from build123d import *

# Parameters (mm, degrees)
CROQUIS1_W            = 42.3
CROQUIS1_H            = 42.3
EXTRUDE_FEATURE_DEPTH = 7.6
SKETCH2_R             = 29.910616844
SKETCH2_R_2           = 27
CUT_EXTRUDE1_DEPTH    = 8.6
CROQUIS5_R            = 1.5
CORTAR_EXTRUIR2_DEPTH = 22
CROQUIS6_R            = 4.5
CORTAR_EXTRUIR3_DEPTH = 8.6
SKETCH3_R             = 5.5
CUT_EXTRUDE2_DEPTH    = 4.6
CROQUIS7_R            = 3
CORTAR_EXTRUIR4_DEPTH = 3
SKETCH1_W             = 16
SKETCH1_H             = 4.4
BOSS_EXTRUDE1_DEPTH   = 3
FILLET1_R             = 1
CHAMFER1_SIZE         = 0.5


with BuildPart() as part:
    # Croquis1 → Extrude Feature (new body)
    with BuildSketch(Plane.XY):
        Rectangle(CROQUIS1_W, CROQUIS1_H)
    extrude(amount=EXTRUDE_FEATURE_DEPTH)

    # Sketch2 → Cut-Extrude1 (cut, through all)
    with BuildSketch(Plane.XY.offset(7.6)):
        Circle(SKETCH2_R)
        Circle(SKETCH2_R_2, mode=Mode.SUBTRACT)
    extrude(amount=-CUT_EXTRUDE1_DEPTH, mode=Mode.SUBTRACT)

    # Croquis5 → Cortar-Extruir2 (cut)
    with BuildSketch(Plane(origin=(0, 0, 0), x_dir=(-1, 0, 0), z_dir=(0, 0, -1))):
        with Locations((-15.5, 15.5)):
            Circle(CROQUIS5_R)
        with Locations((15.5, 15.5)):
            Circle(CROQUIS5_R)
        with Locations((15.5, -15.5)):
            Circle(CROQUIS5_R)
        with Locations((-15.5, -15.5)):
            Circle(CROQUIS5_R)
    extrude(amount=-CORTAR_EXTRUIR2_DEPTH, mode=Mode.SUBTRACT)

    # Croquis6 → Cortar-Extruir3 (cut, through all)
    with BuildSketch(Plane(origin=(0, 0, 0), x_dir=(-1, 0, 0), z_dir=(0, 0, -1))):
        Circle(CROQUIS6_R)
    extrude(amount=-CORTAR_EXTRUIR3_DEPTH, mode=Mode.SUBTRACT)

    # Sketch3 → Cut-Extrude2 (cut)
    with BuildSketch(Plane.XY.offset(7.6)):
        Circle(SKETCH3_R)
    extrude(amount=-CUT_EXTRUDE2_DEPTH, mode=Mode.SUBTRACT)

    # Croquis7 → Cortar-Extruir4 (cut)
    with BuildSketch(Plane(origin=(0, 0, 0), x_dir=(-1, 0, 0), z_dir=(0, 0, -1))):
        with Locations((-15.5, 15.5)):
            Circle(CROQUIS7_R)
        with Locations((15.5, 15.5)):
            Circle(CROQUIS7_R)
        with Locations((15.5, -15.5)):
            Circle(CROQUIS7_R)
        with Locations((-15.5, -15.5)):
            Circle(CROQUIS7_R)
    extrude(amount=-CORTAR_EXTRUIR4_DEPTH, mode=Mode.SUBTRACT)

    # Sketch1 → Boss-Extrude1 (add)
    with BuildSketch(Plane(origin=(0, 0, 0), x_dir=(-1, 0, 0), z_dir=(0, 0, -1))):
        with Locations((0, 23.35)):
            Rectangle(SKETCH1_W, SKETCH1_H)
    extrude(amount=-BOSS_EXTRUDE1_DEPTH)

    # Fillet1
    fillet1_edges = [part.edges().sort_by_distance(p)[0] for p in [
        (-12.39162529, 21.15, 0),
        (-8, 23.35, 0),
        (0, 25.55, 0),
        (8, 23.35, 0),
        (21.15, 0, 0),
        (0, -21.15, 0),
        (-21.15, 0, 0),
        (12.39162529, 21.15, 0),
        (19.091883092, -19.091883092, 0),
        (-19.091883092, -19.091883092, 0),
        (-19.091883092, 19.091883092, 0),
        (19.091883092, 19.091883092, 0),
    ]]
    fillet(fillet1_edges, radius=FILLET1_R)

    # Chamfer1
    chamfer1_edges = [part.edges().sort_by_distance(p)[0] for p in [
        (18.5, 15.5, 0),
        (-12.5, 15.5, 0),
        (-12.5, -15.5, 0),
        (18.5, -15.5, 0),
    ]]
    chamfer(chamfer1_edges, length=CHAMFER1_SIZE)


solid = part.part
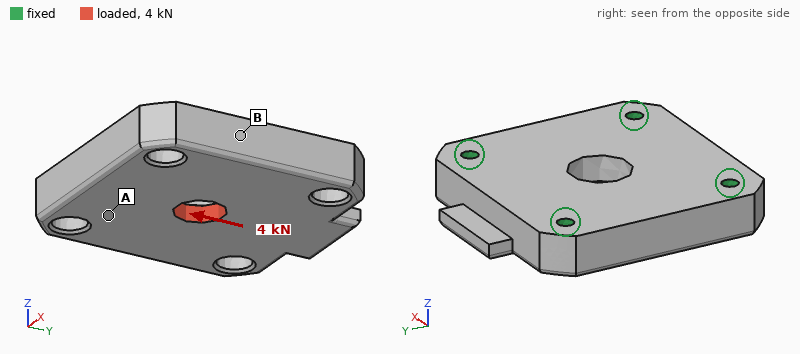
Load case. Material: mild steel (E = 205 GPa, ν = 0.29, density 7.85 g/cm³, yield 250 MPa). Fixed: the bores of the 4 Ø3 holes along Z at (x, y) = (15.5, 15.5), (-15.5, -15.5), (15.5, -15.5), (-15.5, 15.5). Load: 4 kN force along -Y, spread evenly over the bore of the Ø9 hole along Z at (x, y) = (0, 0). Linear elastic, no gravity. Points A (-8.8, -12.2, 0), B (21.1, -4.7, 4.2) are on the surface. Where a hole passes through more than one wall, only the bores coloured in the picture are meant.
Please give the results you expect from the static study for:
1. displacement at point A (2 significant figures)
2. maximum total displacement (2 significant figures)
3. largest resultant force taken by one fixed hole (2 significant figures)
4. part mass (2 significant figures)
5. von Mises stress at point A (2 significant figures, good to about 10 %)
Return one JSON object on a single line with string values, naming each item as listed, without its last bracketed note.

{"displacement at point A": "1.2 µm", "maximum total displacement": "3.0 µm", "largest resultant force taken by one fixed hole": "1.1 kN", "part mass": "97 g", "von Mises stress at point A": "15 MPa"}
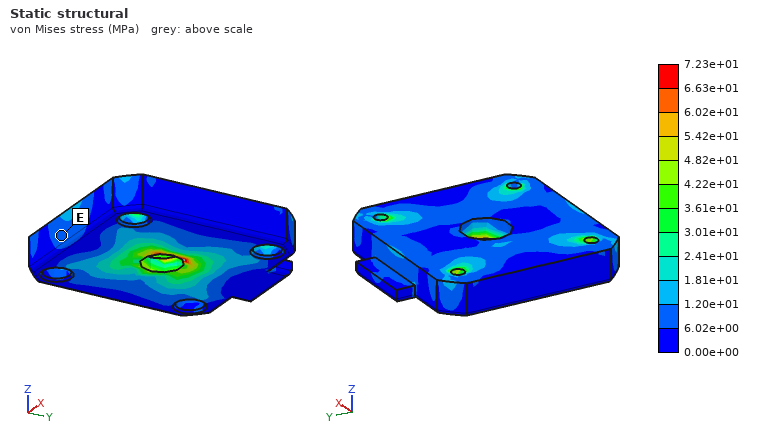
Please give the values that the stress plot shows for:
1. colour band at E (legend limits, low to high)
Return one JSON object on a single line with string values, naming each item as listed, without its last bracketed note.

{"colour band at E": "6.02e+00 to 1.20e+01 MPa"}
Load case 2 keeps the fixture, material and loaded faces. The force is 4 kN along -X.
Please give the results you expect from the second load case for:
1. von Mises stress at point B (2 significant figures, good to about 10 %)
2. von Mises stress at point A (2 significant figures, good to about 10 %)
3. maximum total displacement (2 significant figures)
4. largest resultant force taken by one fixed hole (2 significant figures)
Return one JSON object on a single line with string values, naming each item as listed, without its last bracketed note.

{"von Mises stress at point B": "9.8 MPa", "von Mises stress at point A": "13 MPa", "maximum total displacement": "3.0 µm", "largest resultant force taken by one fixed hole": "1.1 kN"}
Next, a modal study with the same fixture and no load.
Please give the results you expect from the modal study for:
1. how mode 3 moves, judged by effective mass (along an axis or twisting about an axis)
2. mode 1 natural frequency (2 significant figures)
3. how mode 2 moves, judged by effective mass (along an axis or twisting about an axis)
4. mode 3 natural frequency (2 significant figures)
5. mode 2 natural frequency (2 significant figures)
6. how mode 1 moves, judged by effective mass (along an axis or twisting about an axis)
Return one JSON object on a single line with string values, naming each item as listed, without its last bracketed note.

{"how mode 3 moves, judged by effective mass": "twisting about X", "mode 1 natural frequency": "19 kHz", "how mode 2 moves, judged by effective mass": "twisting about X", "mode 3 natural frequency": "27 kHz", "mode 2 natural frequency": "24 kHz", "how mode 1 moves, judged by effective mass": "along Z"}
